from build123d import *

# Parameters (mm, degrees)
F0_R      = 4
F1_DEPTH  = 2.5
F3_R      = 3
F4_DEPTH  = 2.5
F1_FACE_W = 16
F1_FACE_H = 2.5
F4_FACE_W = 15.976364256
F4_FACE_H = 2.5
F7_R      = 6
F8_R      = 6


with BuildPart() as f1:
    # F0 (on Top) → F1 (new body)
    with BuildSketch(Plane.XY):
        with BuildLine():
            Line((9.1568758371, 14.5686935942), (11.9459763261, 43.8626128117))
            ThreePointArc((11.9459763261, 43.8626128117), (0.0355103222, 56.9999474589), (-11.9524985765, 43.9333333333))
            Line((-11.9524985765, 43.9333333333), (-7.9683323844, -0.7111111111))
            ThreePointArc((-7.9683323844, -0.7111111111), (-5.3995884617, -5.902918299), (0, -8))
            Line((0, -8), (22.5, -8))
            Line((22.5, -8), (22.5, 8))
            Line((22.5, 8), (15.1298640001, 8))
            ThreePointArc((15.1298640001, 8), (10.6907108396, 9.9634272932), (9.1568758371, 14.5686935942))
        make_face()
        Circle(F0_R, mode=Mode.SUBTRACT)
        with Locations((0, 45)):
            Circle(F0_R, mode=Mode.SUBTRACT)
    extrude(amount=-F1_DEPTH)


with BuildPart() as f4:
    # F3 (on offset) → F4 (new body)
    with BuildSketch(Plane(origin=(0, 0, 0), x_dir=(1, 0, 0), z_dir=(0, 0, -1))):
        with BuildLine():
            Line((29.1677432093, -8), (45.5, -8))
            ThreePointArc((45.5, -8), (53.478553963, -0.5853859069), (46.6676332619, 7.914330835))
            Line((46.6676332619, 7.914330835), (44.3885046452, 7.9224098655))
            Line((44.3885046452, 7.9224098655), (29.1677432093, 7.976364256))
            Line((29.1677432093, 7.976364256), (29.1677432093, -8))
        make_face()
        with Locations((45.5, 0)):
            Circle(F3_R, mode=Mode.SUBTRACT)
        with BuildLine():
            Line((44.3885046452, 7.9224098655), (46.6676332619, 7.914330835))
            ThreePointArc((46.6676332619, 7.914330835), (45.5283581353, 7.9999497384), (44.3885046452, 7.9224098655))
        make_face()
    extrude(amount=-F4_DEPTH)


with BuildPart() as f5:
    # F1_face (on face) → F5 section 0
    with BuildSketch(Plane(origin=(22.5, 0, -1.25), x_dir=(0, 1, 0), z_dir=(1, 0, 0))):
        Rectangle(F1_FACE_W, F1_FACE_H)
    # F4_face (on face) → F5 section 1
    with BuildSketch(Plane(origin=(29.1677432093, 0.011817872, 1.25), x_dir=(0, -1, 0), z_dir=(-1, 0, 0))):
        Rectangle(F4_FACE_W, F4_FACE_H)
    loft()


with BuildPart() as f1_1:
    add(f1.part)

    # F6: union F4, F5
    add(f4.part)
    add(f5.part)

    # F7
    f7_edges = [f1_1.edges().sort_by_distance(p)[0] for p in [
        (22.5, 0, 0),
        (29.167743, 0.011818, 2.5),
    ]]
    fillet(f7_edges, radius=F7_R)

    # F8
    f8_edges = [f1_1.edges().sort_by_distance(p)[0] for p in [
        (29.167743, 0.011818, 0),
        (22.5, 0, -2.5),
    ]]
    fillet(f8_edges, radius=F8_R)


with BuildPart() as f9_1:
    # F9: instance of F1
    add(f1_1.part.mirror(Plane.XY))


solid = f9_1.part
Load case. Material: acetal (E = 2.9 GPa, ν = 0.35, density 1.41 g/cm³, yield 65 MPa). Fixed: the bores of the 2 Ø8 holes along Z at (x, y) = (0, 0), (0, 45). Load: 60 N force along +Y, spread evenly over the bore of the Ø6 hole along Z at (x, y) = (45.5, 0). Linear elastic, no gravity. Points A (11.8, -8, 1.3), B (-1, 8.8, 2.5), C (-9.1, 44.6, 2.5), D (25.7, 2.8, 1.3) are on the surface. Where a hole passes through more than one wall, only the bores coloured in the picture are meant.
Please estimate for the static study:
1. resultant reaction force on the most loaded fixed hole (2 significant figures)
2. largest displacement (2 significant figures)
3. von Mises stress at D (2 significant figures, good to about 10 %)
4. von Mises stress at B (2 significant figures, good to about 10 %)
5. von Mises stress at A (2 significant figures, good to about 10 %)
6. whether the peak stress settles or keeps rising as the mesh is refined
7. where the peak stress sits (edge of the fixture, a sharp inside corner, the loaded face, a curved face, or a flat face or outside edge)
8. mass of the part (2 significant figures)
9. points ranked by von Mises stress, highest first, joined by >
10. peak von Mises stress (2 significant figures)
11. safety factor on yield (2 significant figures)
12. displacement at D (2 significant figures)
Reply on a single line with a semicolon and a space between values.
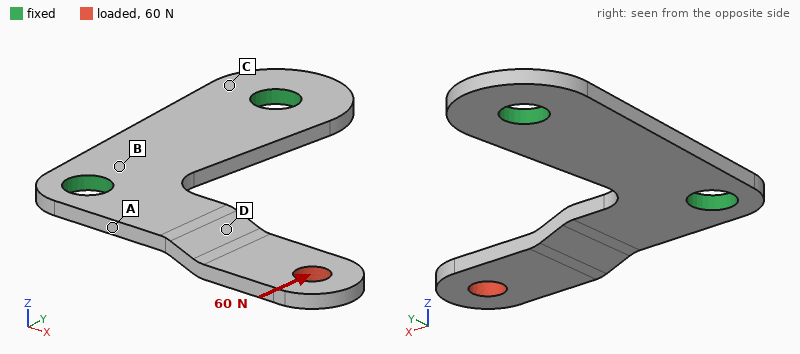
48 N; 1.0 mm; 13 MPa; 5.5 MPa; 17 MPa; settles; a curved face; 6.4 g; A > D > B > C; 30 MPa; 2.1; 0.25 mm
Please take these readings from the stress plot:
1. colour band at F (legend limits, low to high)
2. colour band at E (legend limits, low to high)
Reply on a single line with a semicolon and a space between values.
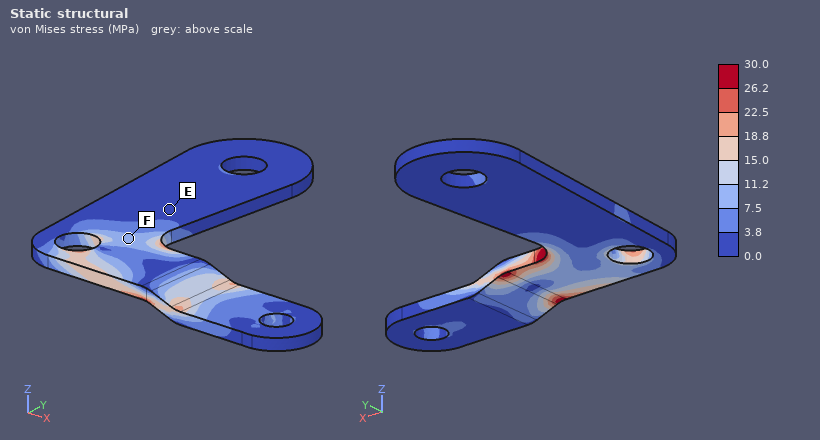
7.5 to 11.2 MPa; 0.0 to 3.8 MPa
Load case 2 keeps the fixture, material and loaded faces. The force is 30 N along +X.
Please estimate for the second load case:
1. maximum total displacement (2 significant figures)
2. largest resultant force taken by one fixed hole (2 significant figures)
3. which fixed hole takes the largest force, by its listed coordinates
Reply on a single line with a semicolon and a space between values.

1.0 mm; 29 N; (0, 0)
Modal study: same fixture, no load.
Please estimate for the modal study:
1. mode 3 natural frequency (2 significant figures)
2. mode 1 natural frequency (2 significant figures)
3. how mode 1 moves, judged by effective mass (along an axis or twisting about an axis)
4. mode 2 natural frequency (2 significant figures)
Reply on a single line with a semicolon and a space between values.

1500 Hz; 270 Hz; along Z; 1400 Hz
